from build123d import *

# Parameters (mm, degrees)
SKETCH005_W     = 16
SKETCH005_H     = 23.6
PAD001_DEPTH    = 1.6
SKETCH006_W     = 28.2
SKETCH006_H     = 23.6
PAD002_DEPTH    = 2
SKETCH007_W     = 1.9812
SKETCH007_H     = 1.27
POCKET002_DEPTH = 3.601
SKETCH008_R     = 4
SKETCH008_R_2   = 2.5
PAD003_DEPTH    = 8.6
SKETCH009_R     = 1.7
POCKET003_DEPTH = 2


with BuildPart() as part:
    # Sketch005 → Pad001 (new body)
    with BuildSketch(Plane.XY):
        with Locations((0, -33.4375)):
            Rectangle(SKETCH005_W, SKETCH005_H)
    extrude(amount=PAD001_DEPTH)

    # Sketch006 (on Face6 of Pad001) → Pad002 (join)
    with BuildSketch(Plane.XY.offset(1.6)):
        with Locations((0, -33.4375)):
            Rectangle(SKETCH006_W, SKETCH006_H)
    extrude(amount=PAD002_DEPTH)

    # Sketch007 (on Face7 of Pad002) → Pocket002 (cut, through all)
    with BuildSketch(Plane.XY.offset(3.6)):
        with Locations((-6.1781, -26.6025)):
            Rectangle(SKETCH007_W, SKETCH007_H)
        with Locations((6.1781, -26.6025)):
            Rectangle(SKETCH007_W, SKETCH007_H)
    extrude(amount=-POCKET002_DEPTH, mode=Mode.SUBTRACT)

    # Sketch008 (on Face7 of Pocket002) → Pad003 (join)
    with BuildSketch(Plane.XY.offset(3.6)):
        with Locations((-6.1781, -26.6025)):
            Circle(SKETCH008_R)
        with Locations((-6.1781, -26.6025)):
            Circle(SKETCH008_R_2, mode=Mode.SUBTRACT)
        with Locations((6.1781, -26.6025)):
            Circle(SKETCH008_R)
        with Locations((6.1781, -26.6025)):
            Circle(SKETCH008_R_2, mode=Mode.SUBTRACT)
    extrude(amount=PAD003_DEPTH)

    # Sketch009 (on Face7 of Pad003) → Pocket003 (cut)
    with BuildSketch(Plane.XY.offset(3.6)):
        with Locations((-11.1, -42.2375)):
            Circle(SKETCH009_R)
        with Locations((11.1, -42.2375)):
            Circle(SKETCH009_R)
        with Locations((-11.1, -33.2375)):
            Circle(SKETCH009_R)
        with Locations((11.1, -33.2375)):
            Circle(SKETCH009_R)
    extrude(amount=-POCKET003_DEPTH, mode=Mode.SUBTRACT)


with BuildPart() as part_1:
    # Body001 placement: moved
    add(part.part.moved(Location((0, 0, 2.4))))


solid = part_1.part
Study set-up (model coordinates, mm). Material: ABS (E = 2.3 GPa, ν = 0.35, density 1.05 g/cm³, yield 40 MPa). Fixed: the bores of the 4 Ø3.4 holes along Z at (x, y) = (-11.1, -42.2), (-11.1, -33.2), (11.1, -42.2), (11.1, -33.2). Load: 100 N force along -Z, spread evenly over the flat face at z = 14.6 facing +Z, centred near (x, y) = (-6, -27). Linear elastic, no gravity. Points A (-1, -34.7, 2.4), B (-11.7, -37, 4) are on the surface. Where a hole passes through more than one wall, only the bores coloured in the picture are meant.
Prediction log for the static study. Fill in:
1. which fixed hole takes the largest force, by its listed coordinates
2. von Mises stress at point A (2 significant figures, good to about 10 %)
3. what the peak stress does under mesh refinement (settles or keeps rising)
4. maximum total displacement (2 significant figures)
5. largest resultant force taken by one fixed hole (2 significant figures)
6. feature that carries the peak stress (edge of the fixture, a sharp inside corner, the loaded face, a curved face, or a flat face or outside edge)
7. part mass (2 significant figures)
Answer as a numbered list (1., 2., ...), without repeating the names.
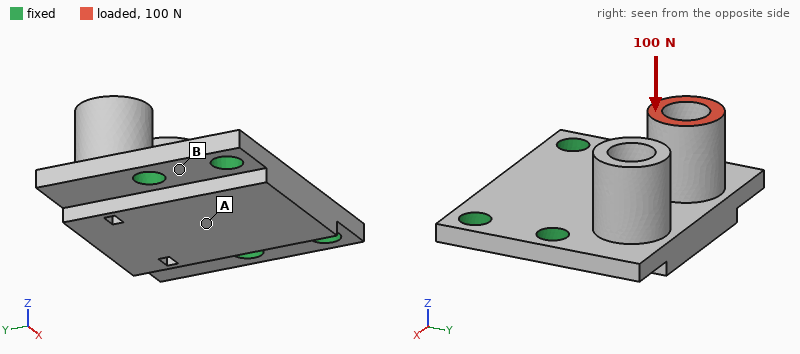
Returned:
1. (-11.1, -33.2)
2. 7.6 MPa
3. keeps rising
4. 0.40 mm
5. 110 N
6. edge of the fixture
7. 2.5 g
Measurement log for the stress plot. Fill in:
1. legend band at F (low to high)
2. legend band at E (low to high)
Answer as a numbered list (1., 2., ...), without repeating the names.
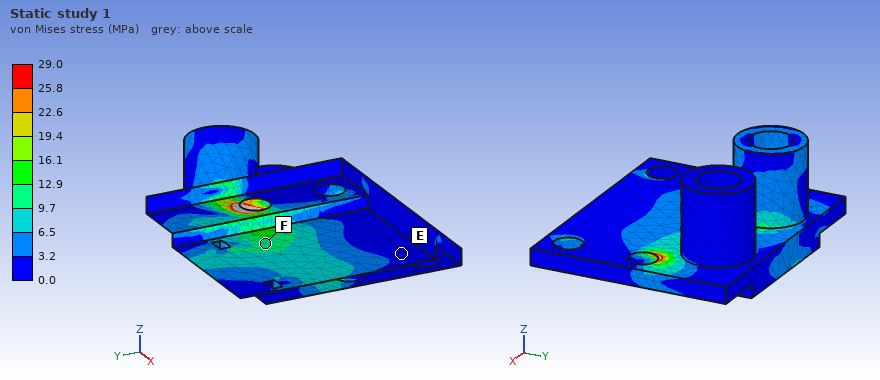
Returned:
1. 9.7 to 12.9 MPa
2. 0.0 to 3.2 MPa
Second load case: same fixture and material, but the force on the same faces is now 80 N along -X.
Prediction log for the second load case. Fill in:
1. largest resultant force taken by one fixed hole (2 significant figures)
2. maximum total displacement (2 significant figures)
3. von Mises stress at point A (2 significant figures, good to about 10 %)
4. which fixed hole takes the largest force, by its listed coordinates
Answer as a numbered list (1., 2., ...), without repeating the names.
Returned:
1. 88 N
2. 0.34 mm
3. 5.6 MPa
4. (-11.1, -33.2)
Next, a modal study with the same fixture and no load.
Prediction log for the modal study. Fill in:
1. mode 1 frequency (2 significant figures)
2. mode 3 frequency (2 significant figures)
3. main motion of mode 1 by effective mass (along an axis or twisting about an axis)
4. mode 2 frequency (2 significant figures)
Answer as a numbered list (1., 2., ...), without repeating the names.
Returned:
1. 2800 Hz
2. 6300 Hz
3. along Z
4. 5200 Hz
